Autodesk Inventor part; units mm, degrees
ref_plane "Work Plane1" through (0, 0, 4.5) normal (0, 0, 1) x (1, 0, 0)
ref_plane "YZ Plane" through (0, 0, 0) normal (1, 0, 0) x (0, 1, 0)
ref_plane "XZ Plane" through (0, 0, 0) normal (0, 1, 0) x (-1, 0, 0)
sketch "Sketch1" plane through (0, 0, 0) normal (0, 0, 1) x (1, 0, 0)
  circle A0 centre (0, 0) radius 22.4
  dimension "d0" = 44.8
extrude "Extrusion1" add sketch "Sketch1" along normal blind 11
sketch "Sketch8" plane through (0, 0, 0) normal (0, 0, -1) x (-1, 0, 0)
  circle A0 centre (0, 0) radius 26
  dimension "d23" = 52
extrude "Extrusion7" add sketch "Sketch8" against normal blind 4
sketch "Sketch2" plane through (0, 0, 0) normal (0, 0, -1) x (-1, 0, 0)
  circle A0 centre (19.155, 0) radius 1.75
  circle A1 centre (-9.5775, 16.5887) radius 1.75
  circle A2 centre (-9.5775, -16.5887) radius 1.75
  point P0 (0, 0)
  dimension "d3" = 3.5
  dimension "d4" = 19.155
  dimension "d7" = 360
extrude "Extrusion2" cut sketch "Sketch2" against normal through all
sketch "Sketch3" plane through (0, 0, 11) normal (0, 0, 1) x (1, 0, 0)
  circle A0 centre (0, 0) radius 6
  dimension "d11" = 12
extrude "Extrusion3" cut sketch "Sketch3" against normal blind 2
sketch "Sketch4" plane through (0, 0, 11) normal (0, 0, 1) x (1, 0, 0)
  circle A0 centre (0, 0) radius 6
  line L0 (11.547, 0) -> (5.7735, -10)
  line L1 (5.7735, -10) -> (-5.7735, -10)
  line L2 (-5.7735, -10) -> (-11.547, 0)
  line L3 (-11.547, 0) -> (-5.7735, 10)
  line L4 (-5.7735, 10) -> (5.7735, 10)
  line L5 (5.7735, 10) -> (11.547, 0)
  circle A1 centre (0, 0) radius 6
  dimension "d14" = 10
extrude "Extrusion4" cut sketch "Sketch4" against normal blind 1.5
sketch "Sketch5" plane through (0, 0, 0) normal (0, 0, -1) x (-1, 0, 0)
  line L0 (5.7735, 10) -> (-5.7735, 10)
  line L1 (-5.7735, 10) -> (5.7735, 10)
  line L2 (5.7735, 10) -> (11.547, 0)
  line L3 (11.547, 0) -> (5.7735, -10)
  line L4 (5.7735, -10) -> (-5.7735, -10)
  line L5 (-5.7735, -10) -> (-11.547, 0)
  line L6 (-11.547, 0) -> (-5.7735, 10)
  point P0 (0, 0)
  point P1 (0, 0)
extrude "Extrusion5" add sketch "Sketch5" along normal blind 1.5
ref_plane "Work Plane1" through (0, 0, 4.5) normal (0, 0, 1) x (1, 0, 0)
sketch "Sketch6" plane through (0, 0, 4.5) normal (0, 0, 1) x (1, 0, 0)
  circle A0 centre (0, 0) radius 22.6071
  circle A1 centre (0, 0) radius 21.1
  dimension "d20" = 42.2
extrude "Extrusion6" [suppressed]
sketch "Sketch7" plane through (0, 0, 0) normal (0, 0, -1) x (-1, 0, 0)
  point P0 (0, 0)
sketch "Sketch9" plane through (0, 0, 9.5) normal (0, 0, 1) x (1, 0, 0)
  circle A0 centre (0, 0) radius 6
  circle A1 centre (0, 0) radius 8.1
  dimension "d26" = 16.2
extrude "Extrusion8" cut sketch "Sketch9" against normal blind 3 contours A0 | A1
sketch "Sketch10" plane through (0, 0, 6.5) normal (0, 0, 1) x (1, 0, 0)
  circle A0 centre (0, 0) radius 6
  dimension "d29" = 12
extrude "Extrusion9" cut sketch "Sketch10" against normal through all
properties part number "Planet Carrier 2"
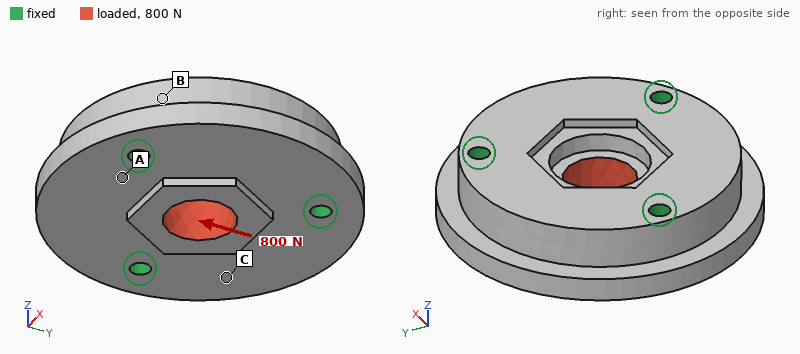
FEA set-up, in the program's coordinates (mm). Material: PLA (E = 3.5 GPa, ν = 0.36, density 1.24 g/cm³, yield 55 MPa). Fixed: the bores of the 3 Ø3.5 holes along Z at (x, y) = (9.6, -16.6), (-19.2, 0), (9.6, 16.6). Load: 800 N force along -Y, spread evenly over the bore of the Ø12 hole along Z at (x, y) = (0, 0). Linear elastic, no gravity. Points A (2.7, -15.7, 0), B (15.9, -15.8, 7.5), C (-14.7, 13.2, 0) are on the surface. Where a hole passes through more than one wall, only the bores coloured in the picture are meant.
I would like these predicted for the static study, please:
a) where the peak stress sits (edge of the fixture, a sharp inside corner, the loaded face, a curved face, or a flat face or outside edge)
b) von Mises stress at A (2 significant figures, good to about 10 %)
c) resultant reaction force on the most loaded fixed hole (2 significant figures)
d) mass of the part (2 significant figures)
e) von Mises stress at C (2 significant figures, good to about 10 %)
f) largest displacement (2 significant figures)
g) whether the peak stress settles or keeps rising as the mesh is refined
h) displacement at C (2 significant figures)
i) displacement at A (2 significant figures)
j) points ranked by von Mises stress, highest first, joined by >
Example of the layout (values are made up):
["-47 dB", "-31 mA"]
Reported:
["edge of the fixture", "2.3 MPa", "270 N", "22 g", "1.2 MPa", "21 µm", "keeps rising", "11 µm", "8.8 µm", "A > C > B"]
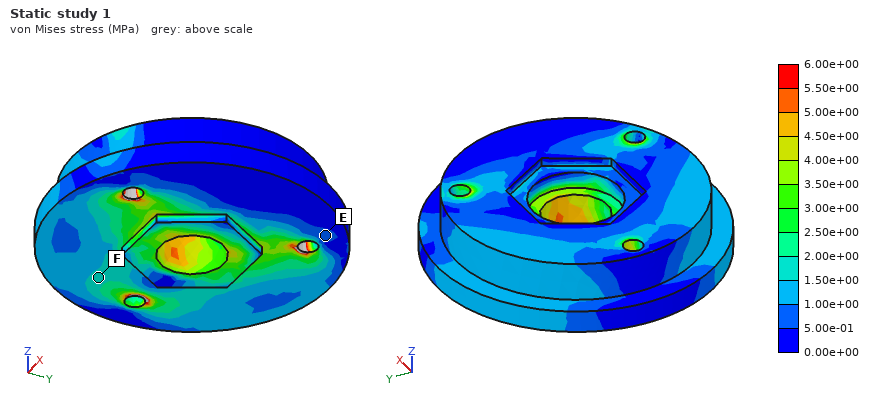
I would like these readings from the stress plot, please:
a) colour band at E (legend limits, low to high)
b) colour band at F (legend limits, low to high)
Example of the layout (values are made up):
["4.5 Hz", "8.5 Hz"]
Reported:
["5.00e-01 to 1.00e+00 MPa", "1.50e+00 to 2.00e+00 MPa"]
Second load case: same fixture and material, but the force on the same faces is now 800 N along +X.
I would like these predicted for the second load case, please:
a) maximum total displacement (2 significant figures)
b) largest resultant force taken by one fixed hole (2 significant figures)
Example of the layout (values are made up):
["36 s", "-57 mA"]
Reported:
["24 µm", "270 N"]
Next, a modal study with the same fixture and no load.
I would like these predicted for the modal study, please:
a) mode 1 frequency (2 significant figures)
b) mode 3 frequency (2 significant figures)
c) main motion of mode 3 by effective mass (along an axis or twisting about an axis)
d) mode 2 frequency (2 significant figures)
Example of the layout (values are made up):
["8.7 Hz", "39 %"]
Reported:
["7200 Hz", "8200 Hz", "along Z", "7200 Hz"]
